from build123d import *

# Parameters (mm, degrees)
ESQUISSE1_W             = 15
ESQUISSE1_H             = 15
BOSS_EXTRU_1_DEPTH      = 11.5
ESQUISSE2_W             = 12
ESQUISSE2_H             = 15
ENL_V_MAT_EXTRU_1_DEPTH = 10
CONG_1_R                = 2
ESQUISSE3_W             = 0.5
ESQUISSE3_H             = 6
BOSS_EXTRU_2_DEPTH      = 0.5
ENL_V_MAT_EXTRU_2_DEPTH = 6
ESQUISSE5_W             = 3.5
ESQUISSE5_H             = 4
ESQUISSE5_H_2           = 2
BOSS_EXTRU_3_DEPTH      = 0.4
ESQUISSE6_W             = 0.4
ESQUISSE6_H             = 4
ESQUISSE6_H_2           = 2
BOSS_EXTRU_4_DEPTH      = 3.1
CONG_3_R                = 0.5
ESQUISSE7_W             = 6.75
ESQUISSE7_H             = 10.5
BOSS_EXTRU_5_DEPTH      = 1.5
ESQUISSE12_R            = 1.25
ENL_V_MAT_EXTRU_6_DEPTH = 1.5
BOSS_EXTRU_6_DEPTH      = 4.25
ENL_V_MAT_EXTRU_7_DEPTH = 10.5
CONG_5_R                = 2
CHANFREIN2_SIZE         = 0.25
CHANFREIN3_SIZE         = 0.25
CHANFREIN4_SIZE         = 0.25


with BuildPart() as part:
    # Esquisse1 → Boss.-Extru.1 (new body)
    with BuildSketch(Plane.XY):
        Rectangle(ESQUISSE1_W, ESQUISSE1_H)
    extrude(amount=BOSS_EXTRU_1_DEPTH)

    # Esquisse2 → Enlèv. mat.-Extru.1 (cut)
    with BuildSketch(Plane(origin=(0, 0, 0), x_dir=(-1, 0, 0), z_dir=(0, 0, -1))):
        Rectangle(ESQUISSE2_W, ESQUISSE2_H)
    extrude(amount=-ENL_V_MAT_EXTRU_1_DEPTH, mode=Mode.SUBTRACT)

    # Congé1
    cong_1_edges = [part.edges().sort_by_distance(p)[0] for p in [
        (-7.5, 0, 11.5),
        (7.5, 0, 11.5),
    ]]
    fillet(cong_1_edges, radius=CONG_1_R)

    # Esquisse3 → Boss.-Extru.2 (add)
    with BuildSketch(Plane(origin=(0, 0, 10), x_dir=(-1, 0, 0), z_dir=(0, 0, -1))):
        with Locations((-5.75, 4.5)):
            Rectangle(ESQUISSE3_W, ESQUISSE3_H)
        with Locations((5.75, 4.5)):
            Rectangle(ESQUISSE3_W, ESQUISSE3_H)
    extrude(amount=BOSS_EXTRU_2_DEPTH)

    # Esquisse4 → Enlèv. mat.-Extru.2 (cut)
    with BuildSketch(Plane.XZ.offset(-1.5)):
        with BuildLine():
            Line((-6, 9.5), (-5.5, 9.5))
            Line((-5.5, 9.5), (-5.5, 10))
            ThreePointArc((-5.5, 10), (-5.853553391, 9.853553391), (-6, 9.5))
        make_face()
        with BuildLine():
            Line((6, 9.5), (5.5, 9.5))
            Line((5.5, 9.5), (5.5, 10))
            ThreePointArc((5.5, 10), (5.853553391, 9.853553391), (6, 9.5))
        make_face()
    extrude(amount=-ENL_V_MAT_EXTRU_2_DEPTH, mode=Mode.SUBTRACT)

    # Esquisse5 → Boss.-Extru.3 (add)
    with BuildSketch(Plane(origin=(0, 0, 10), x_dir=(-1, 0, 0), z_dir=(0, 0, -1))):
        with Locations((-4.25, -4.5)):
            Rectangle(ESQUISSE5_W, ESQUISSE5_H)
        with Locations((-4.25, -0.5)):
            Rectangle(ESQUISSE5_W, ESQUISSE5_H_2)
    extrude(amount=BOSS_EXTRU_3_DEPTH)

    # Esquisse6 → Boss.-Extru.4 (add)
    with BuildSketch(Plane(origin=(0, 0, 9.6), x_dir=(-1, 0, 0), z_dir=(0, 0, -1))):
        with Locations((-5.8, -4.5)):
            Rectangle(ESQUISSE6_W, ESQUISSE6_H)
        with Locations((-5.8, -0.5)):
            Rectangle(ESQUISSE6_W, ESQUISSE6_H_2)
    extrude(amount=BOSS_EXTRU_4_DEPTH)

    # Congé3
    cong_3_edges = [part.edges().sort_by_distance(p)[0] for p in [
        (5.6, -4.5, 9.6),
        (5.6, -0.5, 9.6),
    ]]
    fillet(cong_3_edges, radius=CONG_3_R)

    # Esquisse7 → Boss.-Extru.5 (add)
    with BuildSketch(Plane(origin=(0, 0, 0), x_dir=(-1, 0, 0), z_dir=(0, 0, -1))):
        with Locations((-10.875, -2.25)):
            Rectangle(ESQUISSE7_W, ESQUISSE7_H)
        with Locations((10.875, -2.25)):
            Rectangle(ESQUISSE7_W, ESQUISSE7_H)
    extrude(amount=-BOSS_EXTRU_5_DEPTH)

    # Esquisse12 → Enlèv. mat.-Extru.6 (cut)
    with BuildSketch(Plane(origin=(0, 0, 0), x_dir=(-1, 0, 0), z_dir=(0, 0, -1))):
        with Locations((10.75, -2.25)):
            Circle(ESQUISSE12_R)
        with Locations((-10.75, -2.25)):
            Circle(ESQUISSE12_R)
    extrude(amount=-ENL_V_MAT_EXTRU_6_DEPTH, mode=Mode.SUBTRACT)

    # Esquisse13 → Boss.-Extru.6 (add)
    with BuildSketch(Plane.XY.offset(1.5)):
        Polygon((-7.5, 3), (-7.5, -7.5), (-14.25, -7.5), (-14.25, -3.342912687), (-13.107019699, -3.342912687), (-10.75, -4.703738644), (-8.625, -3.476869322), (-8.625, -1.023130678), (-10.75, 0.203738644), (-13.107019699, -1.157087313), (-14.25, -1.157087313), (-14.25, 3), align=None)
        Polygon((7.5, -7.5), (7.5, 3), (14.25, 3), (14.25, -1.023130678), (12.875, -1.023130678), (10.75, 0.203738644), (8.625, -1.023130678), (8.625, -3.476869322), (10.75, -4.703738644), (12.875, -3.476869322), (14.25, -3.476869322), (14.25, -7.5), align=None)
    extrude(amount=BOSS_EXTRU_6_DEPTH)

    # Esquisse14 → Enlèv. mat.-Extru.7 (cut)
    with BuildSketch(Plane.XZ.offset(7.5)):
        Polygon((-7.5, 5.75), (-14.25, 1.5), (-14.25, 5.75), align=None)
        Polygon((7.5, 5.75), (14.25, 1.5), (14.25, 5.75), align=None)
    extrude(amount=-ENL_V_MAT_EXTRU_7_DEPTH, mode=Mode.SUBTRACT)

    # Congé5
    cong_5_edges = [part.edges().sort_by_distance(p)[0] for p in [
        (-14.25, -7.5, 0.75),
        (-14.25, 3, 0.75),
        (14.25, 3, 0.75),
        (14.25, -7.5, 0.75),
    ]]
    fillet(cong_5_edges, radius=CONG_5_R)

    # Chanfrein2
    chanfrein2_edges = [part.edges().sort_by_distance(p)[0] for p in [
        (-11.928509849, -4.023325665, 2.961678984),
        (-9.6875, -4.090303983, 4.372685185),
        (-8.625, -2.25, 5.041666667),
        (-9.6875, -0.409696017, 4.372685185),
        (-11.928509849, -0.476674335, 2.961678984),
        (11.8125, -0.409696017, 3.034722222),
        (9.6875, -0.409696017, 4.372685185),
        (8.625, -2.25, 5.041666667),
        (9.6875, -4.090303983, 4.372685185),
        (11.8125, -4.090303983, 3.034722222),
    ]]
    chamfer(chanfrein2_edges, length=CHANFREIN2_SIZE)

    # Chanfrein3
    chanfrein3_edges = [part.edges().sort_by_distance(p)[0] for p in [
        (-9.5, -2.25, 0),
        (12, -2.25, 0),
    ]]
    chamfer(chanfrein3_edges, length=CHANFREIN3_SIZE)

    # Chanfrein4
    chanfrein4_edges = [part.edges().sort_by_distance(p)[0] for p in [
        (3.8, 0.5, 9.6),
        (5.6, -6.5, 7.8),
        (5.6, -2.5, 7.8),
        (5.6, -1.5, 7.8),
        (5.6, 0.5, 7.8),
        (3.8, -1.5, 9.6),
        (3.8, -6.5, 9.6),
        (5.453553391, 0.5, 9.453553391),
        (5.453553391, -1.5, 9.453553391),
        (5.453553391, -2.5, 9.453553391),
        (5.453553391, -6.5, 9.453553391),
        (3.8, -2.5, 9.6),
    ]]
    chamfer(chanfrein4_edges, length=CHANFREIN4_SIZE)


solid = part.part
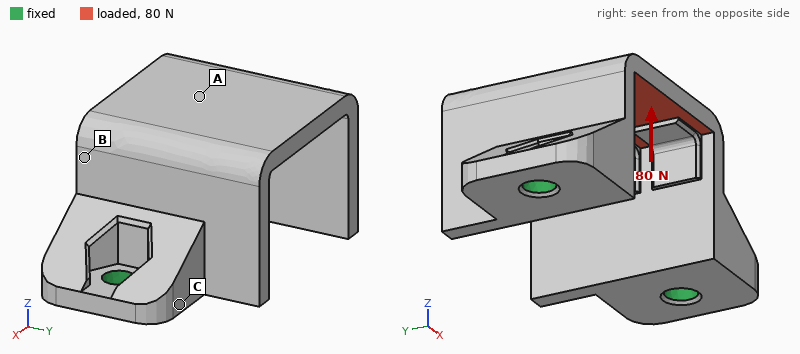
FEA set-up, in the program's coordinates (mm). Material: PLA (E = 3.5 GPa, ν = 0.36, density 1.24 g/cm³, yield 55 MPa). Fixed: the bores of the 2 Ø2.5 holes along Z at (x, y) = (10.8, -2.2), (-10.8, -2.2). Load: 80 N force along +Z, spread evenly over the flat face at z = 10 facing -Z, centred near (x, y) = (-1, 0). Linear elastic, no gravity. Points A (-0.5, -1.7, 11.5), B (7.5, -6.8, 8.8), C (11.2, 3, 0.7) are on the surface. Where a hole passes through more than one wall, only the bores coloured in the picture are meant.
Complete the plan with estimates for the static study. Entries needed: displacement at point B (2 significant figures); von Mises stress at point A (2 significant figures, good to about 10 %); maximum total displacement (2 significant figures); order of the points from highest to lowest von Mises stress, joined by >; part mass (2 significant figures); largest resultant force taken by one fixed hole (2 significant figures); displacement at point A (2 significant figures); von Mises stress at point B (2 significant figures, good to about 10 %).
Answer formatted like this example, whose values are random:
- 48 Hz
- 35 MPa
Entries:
- 0.065 mm
- 11 MPa
- 0.19 mm
- A > B > C
- 1.5 g
- 48 N
- 0.11 mm
- 5.4 MPa
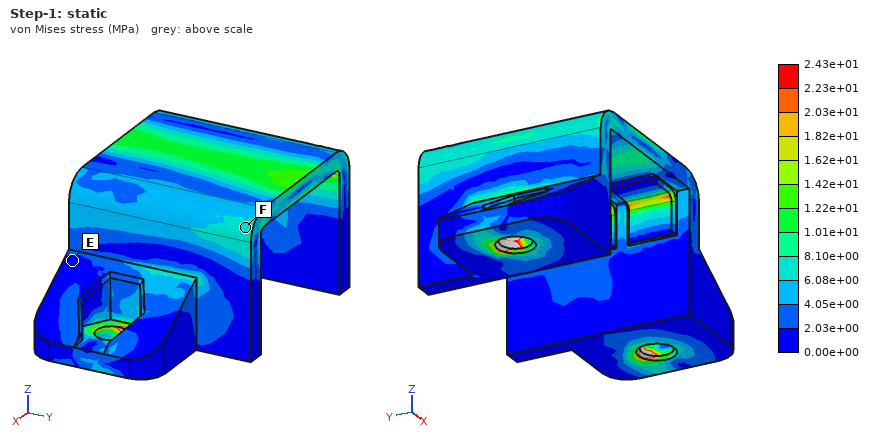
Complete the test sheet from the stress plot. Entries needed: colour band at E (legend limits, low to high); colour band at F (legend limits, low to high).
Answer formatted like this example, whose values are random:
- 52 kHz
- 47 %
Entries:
- 0.00e+00 to 2.03e+00 MPa
- 6.08e+00 to 8.10e+00 MPa
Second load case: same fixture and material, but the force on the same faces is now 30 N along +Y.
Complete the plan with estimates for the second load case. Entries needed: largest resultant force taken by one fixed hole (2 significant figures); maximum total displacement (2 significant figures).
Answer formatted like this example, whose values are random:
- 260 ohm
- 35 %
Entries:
- 16 N
- 0.16 mm
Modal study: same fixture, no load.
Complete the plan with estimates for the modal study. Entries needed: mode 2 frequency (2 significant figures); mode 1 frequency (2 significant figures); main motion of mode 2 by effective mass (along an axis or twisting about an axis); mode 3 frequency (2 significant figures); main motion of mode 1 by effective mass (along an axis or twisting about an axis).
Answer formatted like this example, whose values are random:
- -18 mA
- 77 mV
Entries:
- 4100 Hz
- 2800 Hz
- along X
- 5100 Hz
- along Y
